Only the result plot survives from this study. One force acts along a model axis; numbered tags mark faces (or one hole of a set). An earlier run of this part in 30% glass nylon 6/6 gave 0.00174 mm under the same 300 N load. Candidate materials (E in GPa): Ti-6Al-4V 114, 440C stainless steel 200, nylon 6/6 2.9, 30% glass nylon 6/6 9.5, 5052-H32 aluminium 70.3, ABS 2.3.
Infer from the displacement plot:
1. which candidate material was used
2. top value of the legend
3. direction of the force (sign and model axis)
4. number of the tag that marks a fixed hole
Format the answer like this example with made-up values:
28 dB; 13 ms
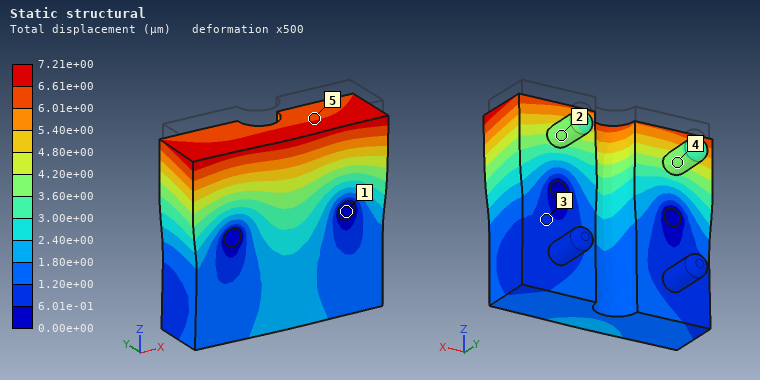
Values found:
ABS; 7.21e+00 µm; -Z; 1
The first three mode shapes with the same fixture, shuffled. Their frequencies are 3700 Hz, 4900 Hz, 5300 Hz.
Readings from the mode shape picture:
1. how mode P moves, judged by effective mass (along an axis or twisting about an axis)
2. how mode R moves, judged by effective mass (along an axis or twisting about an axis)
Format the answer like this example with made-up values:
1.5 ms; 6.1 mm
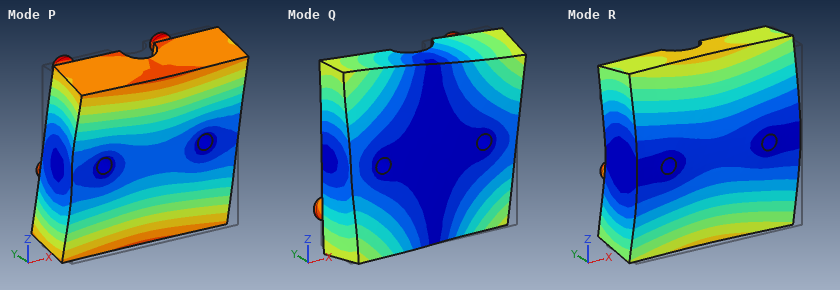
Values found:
twisting about X; along Y
